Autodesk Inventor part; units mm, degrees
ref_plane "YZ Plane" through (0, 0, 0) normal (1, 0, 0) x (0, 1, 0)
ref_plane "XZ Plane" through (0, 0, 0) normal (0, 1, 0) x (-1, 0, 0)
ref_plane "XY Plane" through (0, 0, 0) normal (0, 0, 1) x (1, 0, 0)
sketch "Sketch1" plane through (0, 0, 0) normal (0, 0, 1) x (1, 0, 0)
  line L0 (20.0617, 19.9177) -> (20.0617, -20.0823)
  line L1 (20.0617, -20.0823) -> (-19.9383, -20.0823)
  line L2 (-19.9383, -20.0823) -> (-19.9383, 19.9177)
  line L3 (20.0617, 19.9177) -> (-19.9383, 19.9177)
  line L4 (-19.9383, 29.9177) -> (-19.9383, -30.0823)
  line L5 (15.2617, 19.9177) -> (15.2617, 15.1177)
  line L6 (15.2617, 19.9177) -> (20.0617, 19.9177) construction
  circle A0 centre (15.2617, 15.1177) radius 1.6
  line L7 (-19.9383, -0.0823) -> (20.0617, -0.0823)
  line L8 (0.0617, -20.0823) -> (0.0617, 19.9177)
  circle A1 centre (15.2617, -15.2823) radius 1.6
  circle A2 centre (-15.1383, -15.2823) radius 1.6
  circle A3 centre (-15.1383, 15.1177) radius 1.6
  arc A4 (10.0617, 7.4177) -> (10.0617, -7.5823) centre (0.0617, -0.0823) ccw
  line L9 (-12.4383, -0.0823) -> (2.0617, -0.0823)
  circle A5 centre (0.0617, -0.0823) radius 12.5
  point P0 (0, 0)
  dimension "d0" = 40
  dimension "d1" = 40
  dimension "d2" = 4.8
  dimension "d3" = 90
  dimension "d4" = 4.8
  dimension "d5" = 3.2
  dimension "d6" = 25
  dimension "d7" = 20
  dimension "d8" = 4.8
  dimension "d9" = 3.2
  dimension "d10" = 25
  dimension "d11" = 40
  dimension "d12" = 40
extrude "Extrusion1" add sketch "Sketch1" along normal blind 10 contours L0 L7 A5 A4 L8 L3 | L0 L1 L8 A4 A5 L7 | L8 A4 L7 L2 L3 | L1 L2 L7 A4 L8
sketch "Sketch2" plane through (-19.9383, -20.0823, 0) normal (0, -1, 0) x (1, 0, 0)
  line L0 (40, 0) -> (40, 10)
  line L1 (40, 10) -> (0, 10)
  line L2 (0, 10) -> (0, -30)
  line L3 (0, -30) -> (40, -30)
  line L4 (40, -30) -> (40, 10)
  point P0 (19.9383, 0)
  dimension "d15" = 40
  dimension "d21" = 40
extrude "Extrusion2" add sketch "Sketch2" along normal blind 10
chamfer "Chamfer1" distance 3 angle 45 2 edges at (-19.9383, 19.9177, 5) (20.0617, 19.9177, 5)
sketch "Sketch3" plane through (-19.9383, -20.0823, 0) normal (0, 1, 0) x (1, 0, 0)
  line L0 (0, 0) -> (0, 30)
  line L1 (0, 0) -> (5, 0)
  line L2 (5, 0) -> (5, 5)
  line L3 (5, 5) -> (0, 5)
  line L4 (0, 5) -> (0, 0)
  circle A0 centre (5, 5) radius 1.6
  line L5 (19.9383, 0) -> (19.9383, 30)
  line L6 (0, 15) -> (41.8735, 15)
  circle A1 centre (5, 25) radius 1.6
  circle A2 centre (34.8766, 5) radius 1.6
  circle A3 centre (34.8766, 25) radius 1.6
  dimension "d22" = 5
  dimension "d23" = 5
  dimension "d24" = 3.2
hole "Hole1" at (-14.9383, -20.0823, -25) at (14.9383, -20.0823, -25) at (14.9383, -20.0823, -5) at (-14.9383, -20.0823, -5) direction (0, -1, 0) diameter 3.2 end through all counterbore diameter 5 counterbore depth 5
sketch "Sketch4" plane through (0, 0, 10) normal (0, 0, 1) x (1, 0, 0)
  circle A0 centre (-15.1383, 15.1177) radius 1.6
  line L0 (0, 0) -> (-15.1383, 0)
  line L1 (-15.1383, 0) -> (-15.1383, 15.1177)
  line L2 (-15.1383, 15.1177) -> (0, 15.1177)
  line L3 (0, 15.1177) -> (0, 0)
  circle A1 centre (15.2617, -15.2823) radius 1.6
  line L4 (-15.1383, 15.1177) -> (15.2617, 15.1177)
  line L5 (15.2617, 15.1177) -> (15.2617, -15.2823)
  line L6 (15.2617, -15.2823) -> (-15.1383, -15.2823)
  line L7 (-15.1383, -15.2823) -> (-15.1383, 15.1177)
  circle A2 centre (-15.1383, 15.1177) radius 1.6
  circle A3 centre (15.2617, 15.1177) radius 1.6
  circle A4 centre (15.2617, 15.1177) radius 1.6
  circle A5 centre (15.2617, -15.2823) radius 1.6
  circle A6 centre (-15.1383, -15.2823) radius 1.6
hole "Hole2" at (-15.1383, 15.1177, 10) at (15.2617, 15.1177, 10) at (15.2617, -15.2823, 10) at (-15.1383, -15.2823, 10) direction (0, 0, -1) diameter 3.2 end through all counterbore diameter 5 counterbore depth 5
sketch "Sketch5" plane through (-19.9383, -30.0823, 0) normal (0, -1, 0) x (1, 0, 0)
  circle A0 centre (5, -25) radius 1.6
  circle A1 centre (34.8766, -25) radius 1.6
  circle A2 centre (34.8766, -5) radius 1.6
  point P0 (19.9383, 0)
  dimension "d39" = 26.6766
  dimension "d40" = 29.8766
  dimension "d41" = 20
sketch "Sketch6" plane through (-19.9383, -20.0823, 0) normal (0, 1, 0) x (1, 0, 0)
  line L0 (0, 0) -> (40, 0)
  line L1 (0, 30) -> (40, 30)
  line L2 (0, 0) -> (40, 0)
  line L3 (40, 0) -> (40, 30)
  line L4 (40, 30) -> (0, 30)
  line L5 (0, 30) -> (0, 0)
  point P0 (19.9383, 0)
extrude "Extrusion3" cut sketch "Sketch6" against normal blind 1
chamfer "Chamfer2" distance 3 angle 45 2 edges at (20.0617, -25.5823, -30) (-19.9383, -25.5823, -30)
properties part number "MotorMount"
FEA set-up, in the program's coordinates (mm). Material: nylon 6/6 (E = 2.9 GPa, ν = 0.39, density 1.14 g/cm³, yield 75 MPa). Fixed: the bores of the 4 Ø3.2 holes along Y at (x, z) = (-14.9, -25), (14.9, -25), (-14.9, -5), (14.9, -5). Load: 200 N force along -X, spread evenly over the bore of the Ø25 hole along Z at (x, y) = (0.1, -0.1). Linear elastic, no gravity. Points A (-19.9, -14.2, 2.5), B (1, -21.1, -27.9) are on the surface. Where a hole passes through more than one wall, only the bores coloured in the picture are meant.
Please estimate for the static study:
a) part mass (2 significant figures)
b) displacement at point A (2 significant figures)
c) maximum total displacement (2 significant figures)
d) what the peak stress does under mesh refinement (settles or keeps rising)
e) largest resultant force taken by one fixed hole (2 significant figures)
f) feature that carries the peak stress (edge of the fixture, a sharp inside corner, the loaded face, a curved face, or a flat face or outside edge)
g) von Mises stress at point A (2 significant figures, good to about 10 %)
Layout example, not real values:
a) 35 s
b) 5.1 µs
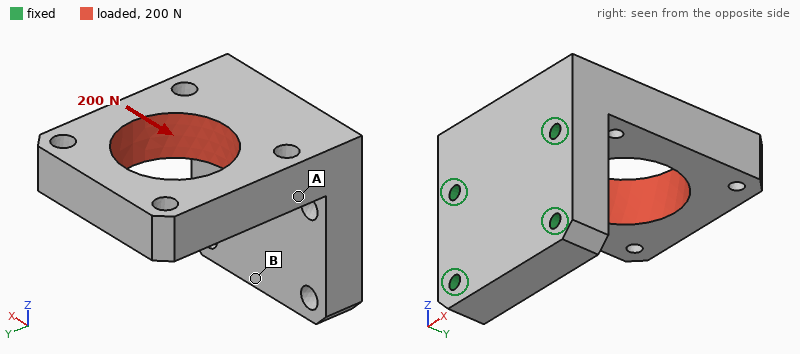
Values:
a) 28 g
b) 0.062 mm
c) 0.19 mm
d) keeps rising
e) 210 N
f) edge of the fixture
g) 3.5 MPa
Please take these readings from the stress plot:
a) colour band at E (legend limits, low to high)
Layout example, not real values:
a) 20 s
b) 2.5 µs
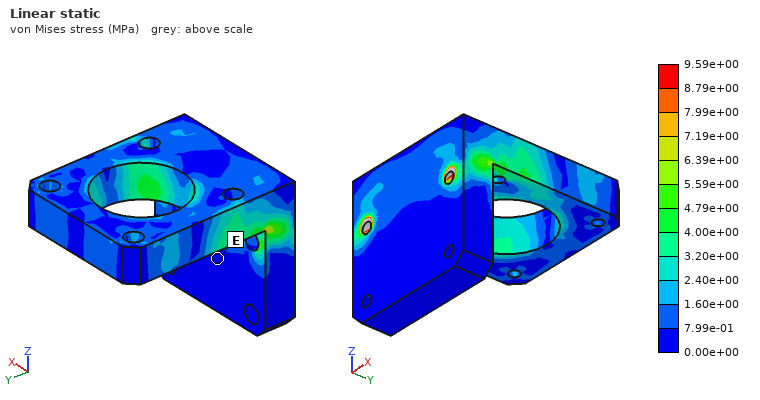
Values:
a) 0.00e+00 to 7.99e-01 MPa
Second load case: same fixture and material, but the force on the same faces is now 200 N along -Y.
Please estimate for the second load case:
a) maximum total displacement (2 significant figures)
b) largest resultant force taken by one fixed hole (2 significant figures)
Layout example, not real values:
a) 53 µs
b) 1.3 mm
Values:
a) 0.16 mm
b) 140 N
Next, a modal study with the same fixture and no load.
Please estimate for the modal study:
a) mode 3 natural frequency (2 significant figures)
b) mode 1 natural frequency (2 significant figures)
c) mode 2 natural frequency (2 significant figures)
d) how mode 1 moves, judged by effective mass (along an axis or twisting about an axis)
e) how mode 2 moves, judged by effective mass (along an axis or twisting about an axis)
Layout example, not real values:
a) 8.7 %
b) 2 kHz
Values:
a) 2300 Hz
b) 810 Hz
c) 1600 Hz
d) along Z
e) along X
